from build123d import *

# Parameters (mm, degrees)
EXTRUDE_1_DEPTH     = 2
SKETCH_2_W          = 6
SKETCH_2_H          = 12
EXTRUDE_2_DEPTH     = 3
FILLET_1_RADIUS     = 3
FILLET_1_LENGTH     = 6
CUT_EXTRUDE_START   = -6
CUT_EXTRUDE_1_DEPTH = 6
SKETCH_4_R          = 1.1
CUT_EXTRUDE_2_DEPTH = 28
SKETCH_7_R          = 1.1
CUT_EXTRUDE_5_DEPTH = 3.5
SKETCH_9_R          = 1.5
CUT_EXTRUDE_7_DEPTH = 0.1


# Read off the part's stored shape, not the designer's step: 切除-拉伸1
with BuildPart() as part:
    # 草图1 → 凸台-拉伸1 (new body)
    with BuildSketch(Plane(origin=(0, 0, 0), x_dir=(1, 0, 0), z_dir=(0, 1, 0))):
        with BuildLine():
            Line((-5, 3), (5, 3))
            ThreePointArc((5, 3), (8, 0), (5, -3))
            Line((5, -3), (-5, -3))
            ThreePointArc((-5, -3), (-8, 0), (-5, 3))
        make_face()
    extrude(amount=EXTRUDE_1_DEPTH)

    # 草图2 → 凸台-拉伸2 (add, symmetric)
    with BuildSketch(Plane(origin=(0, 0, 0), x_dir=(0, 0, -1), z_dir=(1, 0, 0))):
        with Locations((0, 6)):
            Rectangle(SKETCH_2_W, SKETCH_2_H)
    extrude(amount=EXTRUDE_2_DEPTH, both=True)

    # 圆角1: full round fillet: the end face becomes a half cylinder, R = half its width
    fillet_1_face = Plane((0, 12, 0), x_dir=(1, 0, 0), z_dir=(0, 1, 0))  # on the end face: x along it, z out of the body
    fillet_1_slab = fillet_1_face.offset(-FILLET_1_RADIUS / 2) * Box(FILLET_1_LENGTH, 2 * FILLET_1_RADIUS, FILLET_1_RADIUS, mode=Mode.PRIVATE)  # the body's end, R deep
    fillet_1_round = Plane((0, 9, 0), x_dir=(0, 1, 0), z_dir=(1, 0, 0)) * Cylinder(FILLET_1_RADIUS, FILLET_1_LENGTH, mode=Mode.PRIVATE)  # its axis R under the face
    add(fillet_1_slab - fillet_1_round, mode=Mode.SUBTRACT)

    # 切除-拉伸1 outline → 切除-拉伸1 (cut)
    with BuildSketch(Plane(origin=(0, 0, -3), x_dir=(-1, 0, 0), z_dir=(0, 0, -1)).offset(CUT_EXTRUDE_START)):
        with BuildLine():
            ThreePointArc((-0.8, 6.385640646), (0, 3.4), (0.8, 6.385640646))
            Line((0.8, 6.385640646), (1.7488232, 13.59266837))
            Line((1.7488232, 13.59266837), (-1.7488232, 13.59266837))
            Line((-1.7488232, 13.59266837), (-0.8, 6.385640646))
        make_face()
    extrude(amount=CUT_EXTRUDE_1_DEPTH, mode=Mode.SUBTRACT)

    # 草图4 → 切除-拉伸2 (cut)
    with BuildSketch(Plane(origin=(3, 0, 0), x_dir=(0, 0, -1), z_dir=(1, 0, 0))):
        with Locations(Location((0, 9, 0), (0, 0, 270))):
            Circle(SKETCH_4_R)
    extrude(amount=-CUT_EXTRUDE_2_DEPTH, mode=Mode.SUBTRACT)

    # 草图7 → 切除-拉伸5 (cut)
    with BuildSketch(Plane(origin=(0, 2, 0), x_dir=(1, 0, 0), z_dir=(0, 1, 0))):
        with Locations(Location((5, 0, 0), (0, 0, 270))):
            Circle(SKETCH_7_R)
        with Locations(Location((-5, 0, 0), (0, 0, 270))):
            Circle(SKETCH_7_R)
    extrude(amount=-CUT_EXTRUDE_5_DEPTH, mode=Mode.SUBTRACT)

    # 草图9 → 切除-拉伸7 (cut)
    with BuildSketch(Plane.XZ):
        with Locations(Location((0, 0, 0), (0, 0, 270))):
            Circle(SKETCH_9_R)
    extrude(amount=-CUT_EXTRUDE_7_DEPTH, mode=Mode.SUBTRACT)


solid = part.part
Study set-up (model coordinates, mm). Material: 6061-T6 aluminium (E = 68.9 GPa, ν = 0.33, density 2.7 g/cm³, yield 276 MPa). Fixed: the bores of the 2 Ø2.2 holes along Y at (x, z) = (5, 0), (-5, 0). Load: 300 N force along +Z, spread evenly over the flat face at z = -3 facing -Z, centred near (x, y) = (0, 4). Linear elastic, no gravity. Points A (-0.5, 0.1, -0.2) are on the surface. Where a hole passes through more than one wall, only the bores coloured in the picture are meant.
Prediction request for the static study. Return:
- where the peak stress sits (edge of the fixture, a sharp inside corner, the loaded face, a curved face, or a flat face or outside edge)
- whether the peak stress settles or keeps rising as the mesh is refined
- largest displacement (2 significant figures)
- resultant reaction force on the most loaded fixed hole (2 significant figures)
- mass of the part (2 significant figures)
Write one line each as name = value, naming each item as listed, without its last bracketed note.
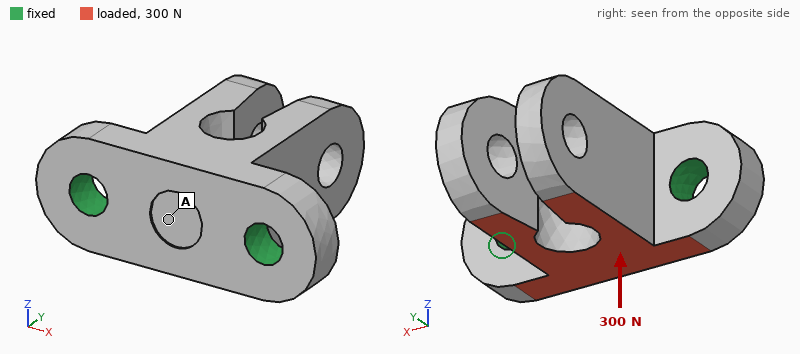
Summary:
where the peak stress sits = edge of the fixture
whether the peak stress settles or keeps rising as the mesh is refined = keeps rising
largest displacement = 24 µm
resultant reaction force on the most loaded fixed hole = 150 N
mass of the part = 1.00 g
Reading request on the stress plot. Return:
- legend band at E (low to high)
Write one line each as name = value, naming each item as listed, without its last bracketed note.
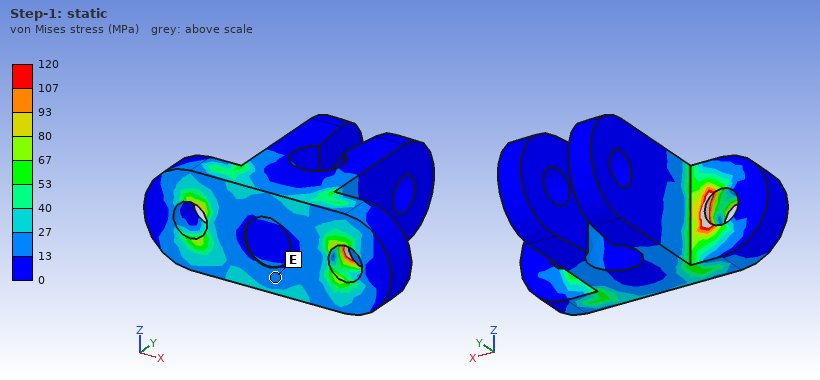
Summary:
legend band at E = 13 to 27 MPa
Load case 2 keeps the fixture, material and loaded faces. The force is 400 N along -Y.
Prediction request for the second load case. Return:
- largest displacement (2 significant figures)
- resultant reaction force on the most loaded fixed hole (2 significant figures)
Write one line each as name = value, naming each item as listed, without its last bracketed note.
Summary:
largest displacement = 31 µm
resultant reaction force on the most loaded fixed hole = 210 N
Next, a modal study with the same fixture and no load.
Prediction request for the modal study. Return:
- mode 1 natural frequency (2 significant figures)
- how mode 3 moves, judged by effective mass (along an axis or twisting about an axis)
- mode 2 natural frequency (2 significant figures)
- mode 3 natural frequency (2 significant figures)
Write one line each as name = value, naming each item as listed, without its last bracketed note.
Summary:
mode 1 natural frequency = 18 kHz
how mode 3 moves, judged by effective mass = along Z
mode 2 natural frequency = 18 kHz
mode 3 natural frequency = 20 kHz
